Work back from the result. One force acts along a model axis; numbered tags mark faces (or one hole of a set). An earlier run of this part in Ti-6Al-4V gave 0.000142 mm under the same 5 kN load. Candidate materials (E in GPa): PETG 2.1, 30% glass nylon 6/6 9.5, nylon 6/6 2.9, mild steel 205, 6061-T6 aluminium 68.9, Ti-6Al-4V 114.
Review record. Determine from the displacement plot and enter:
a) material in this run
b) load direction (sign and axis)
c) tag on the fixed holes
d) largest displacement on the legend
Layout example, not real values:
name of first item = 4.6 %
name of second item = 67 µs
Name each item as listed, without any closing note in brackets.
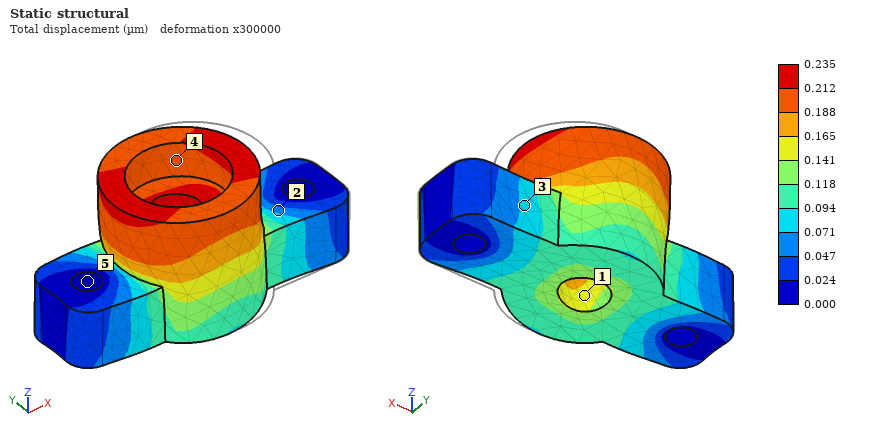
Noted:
material in this run = 6061-T6 aluminium
load direction = -X
tag on the fixed holes = 5
largest displacement on the legend = 0.235 µm
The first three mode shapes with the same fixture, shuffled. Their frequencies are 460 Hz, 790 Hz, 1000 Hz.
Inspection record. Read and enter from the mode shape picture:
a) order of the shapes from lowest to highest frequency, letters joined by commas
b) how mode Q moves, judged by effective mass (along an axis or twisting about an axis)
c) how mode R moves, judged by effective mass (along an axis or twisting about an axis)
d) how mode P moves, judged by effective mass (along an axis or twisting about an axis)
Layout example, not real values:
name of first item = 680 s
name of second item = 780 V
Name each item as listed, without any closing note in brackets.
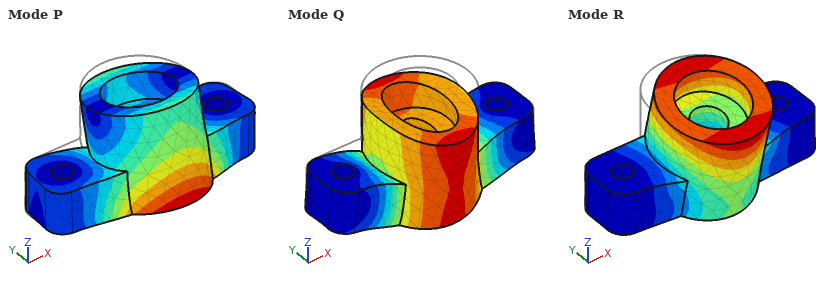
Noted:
order of the shapes from lowest to highest frequency, letters joined by commas = R, Q, P
how mode Q moves, judged by effective mass = along Z
how mode R moves, judged by effective mass = along Y
how mode P moves, judged by effective mass = along Y
